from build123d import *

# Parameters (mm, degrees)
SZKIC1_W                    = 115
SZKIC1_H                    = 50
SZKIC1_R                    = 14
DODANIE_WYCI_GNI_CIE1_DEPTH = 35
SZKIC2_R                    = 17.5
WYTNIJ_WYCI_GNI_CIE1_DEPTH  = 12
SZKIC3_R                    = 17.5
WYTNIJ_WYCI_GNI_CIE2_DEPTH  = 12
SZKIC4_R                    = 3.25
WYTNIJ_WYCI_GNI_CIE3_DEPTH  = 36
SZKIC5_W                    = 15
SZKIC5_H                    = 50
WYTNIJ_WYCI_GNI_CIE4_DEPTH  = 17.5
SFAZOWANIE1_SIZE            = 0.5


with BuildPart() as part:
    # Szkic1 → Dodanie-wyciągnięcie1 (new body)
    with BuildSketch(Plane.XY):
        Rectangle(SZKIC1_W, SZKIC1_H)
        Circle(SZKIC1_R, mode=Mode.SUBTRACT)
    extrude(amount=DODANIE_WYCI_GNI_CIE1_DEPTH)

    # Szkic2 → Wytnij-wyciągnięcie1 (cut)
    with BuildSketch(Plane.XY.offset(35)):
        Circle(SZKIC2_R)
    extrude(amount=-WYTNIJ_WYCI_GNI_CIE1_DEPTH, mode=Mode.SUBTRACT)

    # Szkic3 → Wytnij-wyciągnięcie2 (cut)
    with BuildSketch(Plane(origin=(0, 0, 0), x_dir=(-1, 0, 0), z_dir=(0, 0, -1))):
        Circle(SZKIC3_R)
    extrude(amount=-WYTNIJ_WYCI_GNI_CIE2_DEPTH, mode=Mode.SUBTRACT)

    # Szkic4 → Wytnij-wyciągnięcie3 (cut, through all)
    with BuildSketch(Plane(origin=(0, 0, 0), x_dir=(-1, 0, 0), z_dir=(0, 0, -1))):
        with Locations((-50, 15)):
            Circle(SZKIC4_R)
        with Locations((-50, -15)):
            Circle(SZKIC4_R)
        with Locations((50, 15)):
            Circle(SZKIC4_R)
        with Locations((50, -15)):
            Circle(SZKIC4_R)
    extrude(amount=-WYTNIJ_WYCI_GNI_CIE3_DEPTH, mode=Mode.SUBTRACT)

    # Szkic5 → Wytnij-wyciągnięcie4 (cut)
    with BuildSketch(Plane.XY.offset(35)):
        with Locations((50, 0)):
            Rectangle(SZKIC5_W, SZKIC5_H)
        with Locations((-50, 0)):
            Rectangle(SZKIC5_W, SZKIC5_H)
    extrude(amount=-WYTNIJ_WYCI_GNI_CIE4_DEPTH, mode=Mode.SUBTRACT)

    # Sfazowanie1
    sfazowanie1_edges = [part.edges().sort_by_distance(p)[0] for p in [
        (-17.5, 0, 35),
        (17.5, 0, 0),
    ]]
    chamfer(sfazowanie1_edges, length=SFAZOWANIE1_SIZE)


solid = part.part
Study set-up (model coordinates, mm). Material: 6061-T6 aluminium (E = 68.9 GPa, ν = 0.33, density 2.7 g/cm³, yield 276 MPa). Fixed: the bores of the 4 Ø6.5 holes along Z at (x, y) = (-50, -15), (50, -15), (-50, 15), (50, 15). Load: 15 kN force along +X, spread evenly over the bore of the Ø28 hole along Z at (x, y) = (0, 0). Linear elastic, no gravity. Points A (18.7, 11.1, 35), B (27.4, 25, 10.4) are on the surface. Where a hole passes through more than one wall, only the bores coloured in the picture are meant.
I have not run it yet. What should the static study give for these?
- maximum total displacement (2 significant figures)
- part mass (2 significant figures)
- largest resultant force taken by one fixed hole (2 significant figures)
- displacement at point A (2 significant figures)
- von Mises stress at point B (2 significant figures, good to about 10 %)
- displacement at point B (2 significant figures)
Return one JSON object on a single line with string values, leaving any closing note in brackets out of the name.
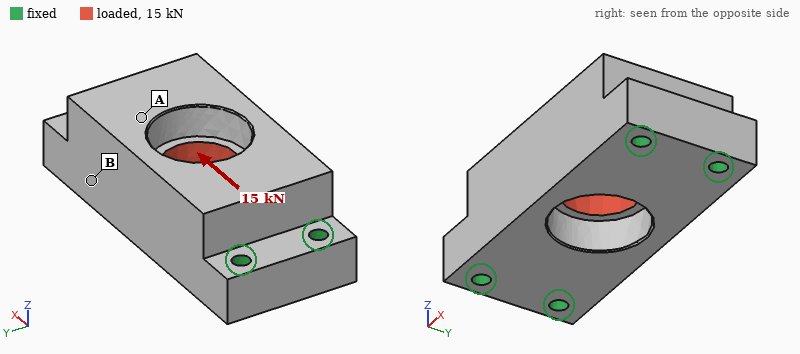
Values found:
{"maximum total displacement": "7.5 µm", "part mass": "390 g", "largest resultant force taken by one fixed hole": "3.8 kN", "displacement at point A": "4.7 µm", "von Mises stress at point B": "7.6 MPa", "displacement at point B": "3.0 µm"}
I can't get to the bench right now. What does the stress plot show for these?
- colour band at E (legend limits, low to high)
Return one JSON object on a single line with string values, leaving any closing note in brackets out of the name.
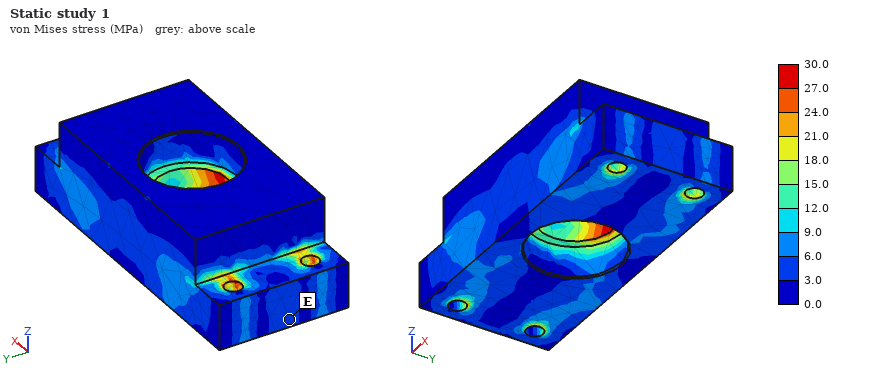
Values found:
{"colour band at E": "3.0 to 6.0 MPa"}
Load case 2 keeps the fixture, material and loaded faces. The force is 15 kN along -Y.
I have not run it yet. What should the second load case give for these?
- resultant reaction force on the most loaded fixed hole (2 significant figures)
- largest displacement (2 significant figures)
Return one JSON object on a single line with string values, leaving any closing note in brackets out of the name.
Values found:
{"resultant reaction force on the most loaded fixed hole": "5.7 kN", "largest displacement": "23 µm"}
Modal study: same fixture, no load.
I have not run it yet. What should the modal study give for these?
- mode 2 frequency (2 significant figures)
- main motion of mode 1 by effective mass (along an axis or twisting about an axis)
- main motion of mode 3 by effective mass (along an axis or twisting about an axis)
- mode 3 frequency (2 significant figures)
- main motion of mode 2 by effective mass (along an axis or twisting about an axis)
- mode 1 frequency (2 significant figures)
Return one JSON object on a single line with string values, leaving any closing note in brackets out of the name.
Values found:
{"mode 2 frequency": "9100 Hz", "main motion of mode 1 by effective mass": "along Z", "main motion of mode 3 by effective mass": "along Y", "mode 3 frequency": "13 kHz", "main motion of mode 2 by effective mass": "along Y", "mode 1 frequency": "8300 Hz"}
